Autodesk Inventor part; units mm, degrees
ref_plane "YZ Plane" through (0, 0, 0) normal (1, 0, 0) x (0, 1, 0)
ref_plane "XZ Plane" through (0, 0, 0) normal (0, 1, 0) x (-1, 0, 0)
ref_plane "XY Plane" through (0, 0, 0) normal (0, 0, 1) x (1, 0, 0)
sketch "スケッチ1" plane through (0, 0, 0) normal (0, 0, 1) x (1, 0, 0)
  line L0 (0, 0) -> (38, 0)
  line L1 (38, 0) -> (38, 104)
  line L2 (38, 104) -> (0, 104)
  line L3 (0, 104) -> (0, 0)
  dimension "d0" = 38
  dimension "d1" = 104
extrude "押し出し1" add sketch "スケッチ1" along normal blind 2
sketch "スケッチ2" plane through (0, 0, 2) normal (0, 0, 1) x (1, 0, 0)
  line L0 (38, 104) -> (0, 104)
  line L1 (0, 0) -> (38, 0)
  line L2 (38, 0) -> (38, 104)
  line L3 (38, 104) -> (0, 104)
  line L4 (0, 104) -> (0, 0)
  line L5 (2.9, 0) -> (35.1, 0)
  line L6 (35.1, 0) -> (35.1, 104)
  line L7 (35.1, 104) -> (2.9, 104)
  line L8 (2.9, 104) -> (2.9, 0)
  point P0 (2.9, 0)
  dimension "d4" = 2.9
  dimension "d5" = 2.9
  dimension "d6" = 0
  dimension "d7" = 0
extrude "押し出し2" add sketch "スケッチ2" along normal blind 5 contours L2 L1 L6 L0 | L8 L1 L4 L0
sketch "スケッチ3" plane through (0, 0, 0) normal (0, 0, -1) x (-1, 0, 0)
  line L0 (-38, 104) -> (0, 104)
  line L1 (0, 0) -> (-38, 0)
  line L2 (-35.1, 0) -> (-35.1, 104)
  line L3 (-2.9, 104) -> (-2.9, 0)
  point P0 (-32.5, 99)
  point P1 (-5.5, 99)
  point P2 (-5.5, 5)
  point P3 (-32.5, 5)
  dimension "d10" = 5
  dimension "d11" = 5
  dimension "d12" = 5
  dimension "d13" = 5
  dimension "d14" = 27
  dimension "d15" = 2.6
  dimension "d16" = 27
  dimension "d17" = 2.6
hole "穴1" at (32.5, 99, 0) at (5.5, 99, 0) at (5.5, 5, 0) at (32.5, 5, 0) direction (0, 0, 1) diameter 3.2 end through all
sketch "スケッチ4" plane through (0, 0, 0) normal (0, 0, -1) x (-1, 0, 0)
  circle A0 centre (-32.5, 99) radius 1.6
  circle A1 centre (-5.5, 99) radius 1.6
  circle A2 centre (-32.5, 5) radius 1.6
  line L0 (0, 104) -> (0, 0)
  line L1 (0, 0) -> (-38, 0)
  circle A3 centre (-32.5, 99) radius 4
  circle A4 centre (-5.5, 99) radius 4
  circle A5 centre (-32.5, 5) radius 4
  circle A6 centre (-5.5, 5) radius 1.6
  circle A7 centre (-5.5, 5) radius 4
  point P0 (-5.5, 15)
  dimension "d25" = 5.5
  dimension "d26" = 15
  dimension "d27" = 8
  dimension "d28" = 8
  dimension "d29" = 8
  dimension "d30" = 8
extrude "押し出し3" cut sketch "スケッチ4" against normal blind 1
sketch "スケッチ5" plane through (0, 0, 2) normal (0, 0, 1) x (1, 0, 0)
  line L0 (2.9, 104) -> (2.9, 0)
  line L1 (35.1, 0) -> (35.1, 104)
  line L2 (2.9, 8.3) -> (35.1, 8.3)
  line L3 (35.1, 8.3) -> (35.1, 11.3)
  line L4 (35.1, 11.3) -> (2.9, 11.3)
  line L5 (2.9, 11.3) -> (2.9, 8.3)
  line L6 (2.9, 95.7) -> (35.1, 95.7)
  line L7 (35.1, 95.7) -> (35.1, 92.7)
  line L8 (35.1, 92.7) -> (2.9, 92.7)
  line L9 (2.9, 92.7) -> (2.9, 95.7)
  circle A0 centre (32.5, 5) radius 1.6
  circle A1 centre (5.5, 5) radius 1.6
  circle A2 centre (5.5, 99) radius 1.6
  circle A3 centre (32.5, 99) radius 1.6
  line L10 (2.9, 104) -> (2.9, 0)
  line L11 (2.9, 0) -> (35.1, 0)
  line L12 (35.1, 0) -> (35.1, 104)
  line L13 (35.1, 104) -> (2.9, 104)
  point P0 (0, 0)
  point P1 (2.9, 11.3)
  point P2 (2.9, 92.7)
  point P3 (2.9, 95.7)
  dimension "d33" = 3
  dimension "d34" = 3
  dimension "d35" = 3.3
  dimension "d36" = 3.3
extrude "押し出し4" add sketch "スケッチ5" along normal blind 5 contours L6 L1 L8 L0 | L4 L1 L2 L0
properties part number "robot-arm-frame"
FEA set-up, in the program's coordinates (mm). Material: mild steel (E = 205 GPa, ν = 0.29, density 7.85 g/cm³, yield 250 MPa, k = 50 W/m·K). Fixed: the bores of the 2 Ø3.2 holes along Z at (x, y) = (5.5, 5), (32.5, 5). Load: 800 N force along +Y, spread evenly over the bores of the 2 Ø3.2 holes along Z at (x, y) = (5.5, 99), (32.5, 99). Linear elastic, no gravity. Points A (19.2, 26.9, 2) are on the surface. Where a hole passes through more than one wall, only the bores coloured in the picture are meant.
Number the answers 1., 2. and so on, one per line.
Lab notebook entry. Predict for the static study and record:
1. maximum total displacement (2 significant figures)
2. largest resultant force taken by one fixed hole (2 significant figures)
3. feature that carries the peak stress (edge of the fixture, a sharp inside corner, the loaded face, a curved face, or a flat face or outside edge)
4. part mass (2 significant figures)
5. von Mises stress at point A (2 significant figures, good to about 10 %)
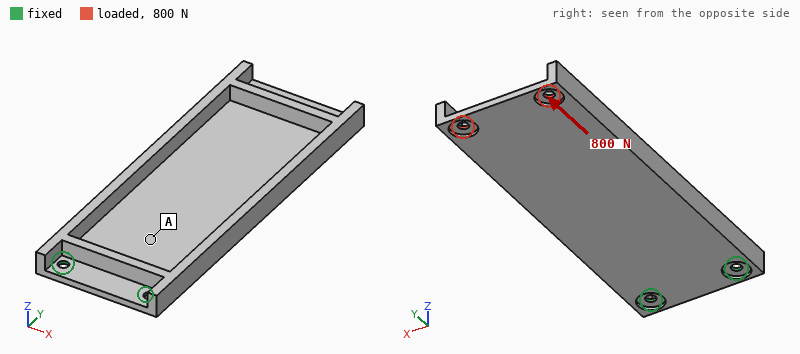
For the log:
1. 30 µm
2. 400 N
3. the loaded face
4. 91 g
5. 6.6 MPa
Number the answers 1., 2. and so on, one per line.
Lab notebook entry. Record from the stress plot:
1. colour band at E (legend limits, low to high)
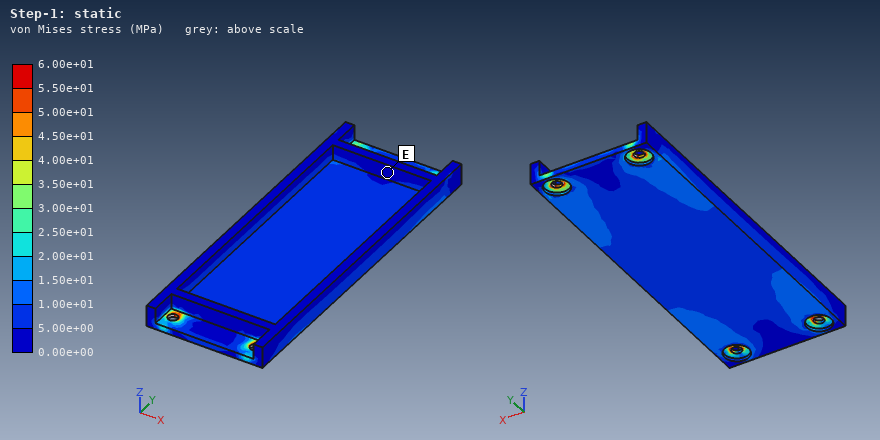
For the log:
1. 0.00e+00 to 5.00e+00 MPa
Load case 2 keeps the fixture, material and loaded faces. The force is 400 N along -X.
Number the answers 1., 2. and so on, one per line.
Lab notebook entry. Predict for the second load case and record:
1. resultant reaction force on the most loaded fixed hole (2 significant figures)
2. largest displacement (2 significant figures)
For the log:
1. 1.4 kN
2. 87 µm
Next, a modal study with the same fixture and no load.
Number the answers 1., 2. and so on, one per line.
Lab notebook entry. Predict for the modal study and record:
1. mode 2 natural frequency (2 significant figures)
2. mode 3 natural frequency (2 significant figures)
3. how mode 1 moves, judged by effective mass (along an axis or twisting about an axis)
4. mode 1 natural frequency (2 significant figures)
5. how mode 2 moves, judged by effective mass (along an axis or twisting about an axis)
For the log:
1. 960 Hz
2. 2300 Hz
3. along Z
4. 260 Hz
5. twisting about Y
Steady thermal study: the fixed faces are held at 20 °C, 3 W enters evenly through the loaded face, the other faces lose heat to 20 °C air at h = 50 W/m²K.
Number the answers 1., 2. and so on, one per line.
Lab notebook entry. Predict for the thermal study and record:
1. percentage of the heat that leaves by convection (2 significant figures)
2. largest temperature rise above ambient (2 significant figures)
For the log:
1. 93 %
2. 20 K
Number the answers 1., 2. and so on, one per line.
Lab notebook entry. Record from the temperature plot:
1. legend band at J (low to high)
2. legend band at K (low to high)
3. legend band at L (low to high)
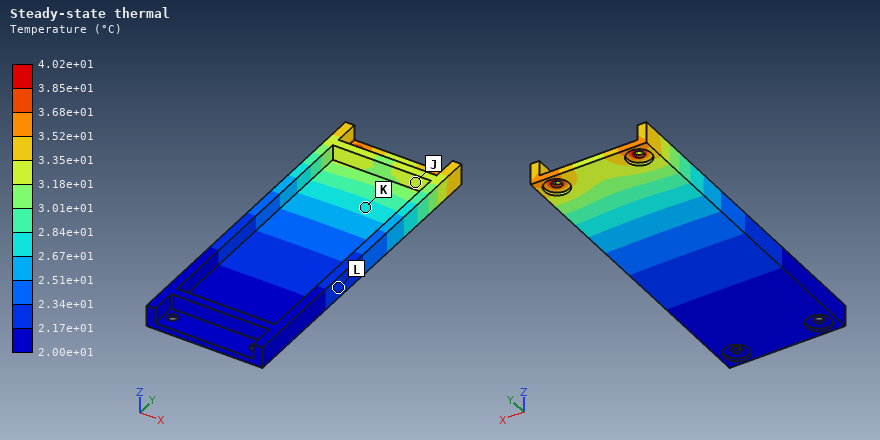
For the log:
1. 3.18e+01 to 3.35e+01 °C
2. 2.67e+01 to 2.84e+01 °C
3. 2.17e+01 to 2.34e+01 °C
